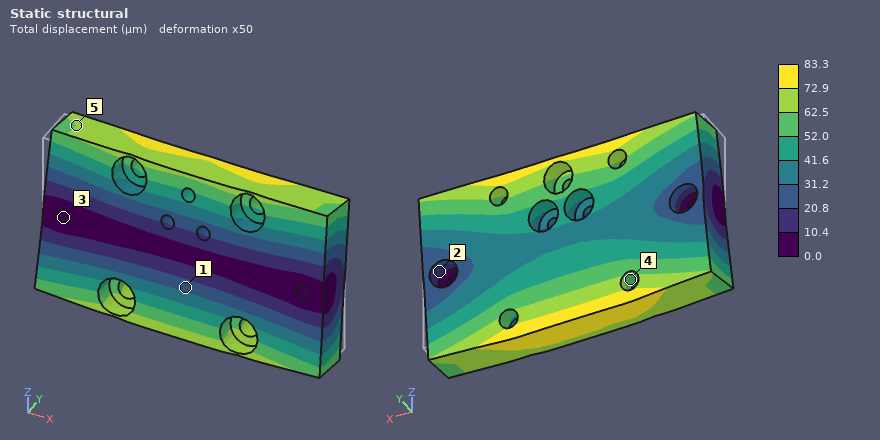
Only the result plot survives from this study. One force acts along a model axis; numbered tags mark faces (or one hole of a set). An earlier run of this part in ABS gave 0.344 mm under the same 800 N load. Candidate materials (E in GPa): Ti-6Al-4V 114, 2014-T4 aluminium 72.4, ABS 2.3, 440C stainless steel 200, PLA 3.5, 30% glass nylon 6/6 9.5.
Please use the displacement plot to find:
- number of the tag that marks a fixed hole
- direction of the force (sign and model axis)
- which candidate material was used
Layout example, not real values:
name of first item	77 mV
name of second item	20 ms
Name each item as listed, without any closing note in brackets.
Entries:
number of the tag that marks a fixed hole	3
direction of the force	-Z
which candidate material was used	30% glass nylon 6/6
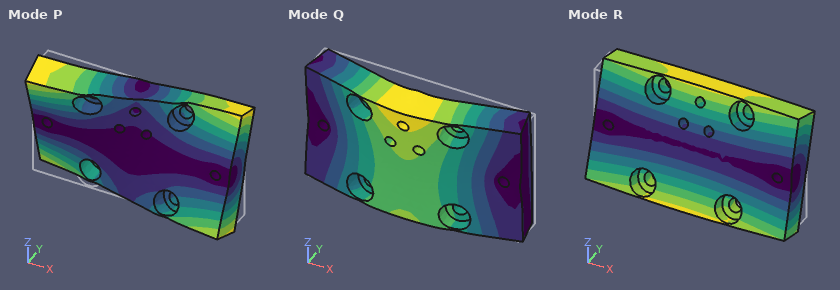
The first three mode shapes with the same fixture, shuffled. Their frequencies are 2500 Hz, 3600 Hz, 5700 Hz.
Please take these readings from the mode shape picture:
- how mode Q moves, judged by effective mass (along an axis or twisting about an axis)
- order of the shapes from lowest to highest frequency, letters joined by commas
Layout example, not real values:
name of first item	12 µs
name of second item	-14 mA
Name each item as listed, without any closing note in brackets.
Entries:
how mode Q moves, judged by effective mass	along Y
order of the shapes from lowest to highest frequency, letters joined by commas	R, Q, P
